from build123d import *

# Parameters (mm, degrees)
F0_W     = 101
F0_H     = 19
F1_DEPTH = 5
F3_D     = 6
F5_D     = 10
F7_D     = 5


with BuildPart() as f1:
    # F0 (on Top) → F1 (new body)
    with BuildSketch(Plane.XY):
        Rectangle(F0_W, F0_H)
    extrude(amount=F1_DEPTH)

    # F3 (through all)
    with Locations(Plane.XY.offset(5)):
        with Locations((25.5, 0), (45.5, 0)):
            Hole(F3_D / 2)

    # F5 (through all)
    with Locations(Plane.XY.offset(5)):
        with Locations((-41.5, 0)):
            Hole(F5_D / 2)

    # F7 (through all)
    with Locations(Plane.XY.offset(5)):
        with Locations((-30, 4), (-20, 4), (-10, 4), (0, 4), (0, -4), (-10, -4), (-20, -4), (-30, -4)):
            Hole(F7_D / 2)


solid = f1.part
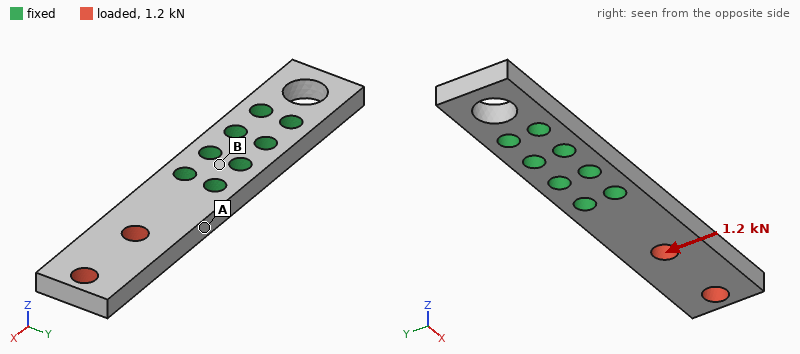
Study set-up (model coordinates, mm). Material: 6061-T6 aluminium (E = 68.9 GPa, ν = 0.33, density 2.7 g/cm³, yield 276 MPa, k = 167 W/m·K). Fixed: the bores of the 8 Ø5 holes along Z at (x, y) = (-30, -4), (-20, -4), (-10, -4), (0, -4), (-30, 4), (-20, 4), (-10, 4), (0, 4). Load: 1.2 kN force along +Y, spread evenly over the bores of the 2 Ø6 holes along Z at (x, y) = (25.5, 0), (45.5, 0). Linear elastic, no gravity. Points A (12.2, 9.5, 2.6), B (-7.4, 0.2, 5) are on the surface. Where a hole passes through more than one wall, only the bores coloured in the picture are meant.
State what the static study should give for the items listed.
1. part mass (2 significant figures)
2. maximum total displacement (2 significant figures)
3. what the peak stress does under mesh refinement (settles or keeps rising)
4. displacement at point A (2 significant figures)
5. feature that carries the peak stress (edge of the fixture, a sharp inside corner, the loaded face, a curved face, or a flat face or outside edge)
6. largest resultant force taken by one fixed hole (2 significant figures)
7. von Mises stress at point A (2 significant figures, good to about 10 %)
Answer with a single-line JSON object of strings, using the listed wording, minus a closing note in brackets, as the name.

{"part mass": "22 g", "maximum total displacement": "0.18 mm", "what the peak stress does under mesh refinement": "keeps rising", "displacement at point A": "0.031 mm", "feature that carries the peak stress": "edge of the fixture", "largest resultant force taken by one fixed hole": "3.2 kN", "von Mises stress at point A": "93 MPa"}
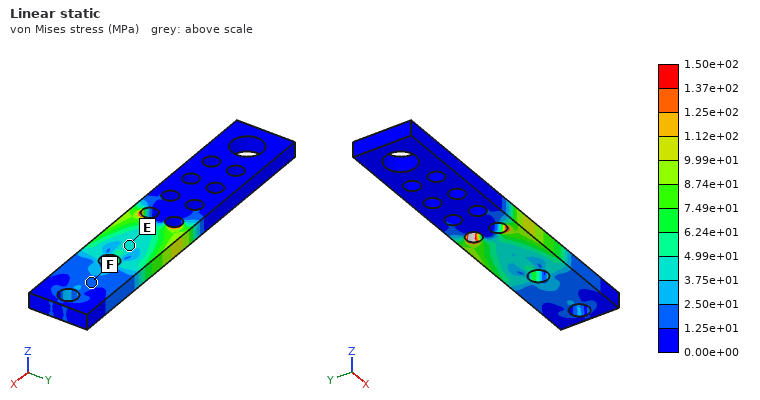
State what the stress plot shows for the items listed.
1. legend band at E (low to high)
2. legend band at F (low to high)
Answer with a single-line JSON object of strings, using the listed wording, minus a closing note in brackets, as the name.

{"legend band at E": "3.75e+01 to 4.99e+01 MPa", "legend band at F": "1.25e+01 to 2.50e+01 MPa"}
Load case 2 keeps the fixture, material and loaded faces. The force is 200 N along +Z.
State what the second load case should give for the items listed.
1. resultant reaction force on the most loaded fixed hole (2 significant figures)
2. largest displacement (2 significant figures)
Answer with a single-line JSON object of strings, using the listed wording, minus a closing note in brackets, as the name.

{"resultant reaction force on the most loaded fixed hole": "120 N", "largest displacement": "0.34 mm"}
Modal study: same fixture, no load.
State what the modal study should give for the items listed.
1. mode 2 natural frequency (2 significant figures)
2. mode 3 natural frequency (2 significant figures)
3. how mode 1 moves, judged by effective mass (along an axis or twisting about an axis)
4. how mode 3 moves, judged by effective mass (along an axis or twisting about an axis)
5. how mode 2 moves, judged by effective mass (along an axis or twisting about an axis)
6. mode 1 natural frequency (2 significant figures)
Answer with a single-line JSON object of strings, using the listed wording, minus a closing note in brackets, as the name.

{"mode 2 natural frequency": "5700 Hz", "mode 3 natural frequency": "7600 Hz", "how mode 1 moves, judged by effective mass": "along Z", "how mode 3 moves, judged by effective mass": "twisting about X", "how mode 2 moves, judged by effective mass": "along Y", "mode 1 natural frequency": "1800 Hz"}
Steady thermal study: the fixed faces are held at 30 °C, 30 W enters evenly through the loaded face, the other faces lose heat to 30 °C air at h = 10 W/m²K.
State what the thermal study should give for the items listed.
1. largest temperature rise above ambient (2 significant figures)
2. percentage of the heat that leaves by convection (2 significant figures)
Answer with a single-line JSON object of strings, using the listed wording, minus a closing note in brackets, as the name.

{"largest temperature rise above ambient": "71 K", "percentage of the heat that leaves by convection": "3.2 %"}
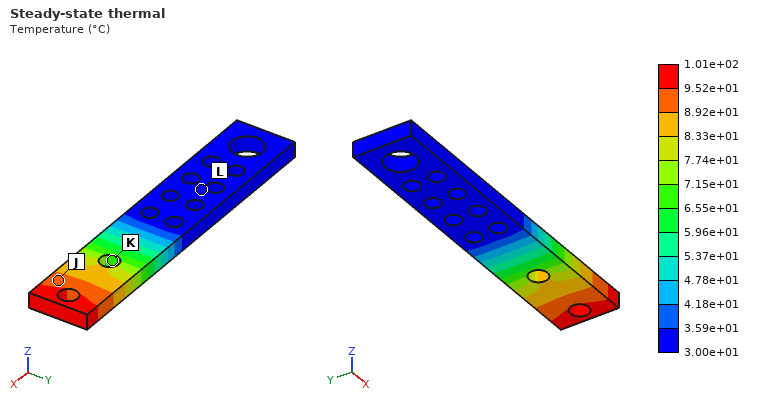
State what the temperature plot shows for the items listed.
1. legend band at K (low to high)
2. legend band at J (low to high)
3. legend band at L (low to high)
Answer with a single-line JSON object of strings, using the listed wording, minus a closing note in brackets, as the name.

{"legend band at K": "6.55e+01 to 7.15e+01 °C", "legend band at J": "8.92e+01 to 9.52e+01 °C", "legend band at L": "3.00e+01 to 3.59e+01 °C"}
